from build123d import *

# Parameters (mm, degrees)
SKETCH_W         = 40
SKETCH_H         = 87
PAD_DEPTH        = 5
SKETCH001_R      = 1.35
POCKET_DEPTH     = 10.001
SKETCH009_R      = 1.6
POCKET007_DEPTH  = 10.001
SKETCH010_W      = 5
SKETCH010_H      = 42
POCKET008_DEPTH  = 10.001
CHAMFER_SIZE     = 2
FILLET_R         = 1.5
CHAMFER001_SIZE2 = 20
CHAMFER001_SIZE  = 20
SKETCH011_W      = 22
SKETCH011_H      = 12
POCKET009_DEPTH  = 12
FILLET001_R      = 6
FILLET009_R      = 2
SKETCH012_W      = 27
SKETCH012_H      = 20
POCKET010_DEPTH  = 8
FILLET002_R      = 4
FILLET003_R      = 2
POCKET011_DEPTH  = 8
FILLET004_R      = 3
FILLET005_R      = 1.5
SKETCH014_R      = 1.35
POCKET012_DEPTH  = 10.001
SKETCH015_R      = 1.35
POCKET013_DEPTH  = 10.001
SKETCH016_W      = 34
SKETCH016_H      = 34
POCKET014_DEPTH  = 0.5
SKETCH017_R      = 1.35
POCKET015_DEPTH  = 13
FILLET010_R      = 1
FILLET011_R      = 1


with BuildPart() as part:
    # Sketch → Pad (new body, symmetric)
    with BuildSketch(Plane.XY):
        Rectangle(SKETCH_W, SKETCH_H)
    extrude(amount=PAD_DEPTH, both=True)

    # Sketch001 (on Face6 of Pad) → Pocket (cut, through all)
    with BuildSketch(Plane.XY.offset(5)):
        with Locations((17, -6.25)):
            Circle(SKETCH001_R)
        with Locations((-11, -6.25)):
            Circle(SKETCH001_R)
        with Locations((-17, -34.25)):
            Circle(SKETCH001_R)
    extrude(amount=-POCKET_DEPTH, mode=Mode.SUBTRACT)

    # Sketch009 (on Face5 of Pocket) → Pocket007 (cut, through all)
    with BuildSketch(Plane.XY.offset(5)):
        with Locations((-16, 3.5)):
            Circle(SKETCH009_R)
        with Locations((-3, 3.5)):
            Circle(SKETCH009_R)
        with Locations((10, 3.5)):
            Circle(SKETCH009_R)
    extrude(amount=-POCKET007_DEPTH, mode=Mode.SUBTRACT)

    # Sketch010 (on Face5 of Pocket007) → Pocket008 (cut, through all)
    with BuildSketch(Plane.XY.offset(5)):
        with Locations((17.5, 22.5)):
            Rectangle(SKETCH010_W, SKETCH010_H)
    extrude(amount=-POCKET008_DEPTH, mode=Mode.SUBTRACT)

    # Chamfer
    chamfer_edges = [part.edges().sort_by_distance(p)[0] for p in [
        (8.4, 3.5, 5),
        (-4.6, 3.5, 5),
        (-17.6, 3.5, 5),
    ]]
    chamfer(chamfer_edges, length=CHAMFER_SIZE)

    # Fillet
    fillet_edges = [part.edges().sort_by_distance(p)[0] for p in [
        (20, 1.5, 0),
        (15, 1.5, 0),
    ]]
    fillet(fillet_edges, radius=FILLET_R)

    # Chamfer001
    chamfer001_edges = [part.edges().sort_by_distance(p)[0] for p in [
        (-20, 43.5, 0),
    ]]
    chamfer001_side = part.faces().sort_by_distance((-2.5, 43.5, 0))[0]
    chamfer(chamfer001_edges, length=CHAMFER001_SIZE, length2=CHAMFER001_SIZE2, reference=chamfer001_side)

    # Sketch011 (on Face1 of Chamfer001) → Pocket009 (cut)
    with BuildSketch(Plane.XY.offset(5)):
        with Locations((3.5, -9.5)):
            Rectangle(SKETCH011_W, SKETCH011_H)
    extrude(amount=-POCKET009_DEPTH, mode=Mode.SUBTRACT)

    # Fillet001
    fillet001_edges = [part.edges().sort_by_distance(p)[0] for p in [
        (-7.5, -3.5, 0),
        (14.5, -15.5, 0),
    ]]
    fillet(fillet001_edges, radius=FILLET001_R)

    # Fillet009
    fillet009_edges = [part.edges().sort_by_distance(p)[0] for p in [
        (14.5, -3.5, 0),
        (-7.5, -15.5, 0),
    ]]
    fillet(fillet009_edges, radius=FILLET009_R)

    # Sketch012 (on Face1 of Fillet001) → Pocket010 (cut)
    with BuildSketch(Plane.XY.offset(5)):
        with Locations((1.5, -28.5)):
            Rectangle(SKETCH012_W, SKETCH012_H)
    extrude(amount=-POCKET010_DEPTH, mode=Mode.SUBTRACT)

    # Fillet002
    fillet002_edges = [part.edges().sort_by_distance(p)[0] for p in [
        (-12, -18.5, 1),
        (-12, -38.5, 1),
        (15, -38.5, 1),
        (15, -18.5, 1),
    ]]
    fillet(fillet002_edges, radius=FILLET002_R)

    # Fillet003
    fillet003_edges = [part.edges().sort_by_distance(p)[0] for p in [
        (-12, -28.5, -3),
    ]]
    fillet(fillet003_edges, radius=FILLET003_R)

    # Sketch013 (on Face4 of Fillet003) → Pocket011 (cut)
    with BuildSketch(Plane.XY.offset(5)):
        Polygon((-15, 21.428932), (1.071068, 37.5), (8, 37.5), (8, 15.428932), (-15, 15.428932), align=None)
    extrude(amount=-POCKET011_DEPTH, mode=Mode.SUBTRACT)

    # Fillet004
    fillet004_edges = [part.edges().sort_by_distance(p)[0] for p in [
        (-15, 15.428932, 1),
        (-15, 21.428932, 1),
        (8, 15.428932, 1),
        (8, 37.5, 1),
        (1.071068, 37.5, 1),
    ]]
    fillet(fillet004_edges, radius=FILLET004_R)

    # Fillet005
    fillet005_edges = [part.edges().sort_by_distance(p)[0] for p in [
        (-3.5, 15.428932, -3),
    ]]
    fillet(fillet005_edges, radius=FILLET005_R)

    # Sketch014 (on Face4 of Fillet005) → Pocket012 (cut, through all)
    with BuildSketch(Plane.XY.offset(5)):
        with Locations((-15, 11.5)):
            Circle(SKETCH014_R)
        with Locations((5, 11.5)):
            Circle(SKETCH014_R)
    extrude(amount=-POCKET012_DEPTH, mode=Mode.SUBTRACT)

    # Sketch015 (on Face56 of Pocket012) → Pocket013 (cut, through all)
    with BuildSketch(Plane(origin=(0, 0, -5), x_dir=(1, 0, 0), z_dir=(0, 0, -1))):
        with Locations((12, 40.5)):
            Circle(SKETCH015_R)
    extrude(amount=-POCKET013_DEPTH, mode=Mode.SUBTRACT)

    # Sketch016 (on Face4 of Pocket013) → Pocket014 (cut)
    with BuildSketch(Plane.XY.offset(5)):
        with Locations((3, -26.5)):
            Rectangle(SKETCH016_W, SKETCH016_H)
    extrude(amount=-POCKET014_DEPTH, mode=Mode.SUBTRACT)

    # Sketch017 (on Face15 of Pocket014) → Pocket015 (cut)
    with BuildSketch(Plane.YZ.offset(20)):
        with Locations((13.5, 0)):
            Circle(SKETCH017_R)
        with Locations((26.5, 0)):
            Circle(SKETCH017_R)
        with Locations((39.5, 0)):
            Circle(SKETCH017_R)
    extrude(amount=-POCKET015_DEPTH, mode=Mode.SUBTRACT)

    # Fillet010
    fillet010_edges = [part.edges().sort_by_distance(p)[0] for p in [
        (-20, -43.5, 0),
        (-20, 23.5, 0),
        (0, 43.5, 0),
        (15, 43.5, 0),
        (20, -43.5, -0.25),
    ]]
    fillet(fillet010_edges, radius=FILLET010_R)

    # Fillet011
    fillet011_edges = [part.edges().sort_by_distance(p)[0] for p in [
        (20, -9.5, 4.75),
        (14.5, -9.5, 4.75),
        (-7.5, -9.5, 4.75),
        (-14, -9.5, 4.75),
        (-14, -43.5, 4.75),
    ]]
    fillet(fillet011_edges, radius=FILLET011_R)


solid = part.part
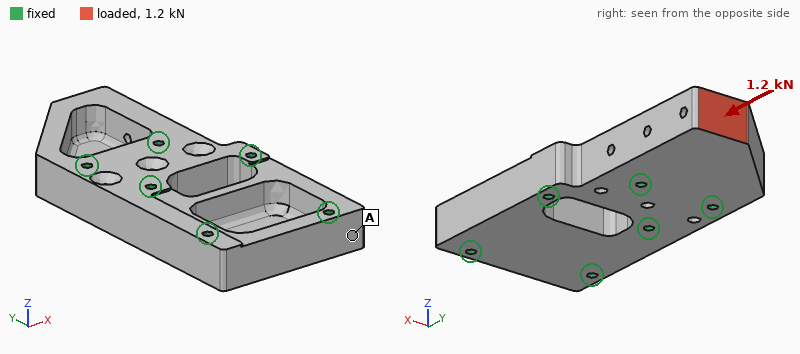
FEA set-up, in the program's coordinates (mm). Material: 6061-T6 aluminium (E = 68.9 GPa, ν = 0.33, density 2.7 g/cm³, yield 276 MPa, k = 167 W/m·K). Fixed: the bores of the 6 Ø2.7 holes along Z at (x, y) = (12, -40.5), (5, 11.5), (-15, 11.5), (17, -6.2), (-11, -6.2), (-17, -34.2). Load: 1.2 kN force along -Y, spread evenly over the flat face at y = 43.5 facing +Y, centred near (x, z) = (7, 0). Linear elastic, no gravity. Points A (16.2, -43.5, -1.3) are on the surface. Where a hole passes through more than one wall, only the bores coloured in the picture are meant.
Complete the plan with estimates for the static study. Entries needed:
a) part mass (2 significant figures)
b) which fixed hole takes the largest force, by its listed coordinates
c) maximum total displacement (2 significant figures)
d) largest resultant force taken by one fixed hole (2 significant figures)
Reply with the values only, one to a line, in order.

54 g
(5, 11.5)
17 µm
860 N
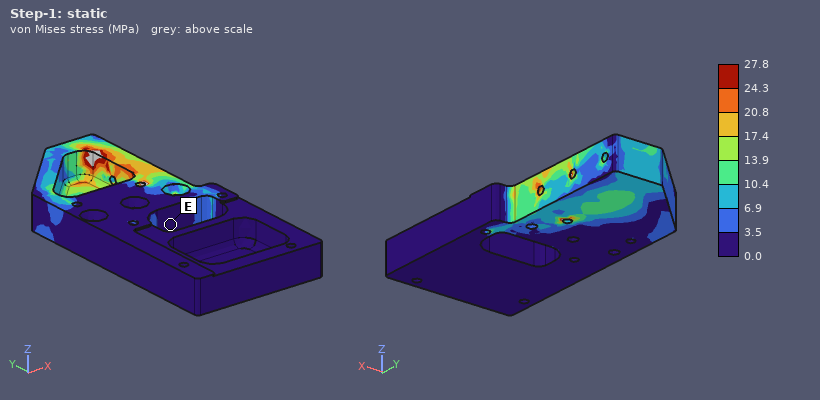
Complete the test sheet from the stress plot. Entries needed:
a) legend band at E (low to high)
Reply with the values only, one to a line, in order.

0.0 to 3.5 MPa
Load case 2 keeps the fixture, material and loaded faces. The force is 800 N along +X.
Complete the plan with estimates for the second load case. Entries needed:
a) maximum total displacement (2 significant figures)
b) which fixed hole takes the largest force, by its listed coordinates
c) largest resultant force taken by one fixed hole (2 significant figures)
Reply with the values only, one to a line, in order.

26 µm
(-15, 11.5)
980 N
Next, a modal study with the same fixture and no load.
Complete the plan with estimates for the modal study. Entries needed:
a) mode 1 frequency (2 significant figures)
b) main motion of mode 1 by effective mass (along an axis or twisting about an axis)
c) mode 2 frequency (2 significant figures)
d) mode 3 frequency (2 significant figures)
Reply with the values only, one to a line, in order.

6300 Hz
along Z
13 kHz
17 kHz
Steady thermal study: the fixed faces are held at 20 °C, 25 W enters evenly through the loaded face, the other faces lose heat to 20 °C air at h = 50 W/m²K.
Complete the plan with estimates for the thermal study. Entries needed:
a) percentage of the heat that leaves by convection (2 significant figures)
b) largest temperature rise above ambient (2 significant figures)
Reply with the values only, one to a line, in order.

9.1 %
34 K
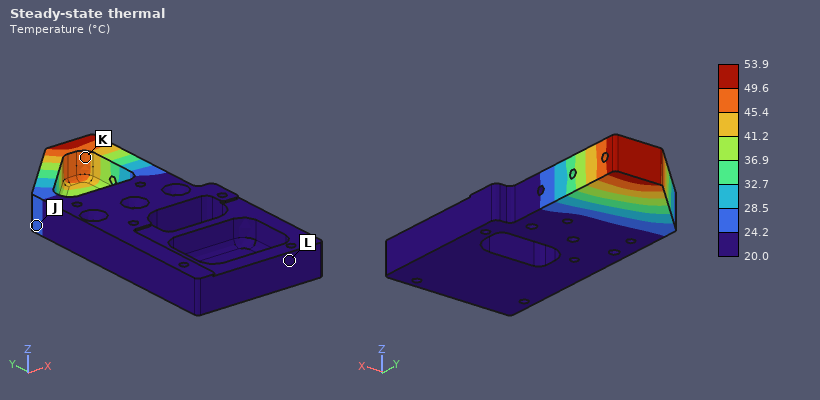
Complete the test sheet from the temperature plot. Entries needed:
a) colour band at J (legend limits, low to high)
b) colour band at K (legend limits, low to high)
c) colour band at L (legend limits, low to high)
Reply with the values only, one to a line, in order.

24.2 to 28.5 °C
45.4 to 49.6 °C
20.0 to 24.2 °C
